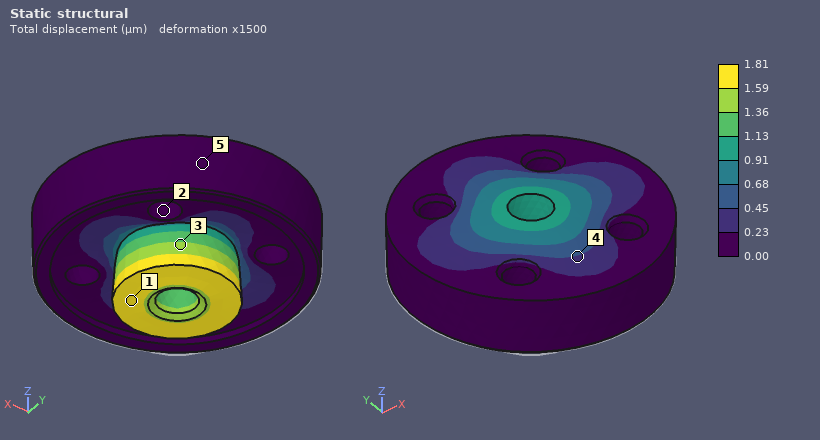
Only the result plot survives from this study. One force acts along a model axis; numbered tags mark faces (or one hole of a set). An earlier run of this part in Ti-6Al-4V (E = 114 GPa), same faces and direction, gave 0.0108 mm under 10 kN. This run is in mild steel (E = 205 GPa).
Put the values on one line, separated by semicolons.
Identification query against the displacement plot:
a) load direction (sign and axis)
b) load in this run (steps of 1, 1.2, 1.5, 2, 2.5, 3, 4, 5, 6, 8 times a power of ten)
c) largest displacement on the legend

+Z; 3 kN; 1.81 µm
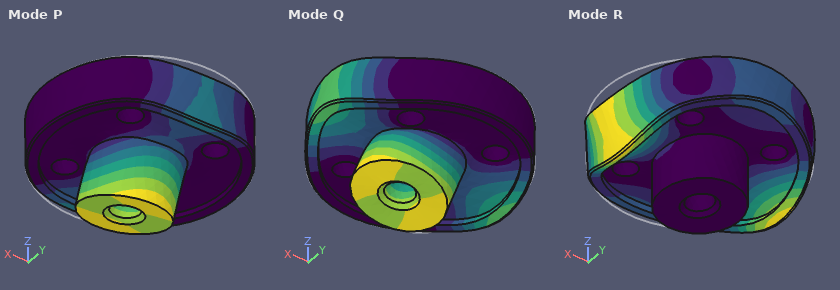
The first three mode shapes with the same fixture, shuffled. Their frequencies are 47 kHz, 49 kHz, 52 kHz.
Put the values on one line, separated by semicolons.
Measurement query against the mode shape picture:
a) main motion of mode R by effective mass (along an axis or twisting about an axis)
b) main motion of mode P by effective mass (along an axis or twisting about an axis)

along Z; along Y
